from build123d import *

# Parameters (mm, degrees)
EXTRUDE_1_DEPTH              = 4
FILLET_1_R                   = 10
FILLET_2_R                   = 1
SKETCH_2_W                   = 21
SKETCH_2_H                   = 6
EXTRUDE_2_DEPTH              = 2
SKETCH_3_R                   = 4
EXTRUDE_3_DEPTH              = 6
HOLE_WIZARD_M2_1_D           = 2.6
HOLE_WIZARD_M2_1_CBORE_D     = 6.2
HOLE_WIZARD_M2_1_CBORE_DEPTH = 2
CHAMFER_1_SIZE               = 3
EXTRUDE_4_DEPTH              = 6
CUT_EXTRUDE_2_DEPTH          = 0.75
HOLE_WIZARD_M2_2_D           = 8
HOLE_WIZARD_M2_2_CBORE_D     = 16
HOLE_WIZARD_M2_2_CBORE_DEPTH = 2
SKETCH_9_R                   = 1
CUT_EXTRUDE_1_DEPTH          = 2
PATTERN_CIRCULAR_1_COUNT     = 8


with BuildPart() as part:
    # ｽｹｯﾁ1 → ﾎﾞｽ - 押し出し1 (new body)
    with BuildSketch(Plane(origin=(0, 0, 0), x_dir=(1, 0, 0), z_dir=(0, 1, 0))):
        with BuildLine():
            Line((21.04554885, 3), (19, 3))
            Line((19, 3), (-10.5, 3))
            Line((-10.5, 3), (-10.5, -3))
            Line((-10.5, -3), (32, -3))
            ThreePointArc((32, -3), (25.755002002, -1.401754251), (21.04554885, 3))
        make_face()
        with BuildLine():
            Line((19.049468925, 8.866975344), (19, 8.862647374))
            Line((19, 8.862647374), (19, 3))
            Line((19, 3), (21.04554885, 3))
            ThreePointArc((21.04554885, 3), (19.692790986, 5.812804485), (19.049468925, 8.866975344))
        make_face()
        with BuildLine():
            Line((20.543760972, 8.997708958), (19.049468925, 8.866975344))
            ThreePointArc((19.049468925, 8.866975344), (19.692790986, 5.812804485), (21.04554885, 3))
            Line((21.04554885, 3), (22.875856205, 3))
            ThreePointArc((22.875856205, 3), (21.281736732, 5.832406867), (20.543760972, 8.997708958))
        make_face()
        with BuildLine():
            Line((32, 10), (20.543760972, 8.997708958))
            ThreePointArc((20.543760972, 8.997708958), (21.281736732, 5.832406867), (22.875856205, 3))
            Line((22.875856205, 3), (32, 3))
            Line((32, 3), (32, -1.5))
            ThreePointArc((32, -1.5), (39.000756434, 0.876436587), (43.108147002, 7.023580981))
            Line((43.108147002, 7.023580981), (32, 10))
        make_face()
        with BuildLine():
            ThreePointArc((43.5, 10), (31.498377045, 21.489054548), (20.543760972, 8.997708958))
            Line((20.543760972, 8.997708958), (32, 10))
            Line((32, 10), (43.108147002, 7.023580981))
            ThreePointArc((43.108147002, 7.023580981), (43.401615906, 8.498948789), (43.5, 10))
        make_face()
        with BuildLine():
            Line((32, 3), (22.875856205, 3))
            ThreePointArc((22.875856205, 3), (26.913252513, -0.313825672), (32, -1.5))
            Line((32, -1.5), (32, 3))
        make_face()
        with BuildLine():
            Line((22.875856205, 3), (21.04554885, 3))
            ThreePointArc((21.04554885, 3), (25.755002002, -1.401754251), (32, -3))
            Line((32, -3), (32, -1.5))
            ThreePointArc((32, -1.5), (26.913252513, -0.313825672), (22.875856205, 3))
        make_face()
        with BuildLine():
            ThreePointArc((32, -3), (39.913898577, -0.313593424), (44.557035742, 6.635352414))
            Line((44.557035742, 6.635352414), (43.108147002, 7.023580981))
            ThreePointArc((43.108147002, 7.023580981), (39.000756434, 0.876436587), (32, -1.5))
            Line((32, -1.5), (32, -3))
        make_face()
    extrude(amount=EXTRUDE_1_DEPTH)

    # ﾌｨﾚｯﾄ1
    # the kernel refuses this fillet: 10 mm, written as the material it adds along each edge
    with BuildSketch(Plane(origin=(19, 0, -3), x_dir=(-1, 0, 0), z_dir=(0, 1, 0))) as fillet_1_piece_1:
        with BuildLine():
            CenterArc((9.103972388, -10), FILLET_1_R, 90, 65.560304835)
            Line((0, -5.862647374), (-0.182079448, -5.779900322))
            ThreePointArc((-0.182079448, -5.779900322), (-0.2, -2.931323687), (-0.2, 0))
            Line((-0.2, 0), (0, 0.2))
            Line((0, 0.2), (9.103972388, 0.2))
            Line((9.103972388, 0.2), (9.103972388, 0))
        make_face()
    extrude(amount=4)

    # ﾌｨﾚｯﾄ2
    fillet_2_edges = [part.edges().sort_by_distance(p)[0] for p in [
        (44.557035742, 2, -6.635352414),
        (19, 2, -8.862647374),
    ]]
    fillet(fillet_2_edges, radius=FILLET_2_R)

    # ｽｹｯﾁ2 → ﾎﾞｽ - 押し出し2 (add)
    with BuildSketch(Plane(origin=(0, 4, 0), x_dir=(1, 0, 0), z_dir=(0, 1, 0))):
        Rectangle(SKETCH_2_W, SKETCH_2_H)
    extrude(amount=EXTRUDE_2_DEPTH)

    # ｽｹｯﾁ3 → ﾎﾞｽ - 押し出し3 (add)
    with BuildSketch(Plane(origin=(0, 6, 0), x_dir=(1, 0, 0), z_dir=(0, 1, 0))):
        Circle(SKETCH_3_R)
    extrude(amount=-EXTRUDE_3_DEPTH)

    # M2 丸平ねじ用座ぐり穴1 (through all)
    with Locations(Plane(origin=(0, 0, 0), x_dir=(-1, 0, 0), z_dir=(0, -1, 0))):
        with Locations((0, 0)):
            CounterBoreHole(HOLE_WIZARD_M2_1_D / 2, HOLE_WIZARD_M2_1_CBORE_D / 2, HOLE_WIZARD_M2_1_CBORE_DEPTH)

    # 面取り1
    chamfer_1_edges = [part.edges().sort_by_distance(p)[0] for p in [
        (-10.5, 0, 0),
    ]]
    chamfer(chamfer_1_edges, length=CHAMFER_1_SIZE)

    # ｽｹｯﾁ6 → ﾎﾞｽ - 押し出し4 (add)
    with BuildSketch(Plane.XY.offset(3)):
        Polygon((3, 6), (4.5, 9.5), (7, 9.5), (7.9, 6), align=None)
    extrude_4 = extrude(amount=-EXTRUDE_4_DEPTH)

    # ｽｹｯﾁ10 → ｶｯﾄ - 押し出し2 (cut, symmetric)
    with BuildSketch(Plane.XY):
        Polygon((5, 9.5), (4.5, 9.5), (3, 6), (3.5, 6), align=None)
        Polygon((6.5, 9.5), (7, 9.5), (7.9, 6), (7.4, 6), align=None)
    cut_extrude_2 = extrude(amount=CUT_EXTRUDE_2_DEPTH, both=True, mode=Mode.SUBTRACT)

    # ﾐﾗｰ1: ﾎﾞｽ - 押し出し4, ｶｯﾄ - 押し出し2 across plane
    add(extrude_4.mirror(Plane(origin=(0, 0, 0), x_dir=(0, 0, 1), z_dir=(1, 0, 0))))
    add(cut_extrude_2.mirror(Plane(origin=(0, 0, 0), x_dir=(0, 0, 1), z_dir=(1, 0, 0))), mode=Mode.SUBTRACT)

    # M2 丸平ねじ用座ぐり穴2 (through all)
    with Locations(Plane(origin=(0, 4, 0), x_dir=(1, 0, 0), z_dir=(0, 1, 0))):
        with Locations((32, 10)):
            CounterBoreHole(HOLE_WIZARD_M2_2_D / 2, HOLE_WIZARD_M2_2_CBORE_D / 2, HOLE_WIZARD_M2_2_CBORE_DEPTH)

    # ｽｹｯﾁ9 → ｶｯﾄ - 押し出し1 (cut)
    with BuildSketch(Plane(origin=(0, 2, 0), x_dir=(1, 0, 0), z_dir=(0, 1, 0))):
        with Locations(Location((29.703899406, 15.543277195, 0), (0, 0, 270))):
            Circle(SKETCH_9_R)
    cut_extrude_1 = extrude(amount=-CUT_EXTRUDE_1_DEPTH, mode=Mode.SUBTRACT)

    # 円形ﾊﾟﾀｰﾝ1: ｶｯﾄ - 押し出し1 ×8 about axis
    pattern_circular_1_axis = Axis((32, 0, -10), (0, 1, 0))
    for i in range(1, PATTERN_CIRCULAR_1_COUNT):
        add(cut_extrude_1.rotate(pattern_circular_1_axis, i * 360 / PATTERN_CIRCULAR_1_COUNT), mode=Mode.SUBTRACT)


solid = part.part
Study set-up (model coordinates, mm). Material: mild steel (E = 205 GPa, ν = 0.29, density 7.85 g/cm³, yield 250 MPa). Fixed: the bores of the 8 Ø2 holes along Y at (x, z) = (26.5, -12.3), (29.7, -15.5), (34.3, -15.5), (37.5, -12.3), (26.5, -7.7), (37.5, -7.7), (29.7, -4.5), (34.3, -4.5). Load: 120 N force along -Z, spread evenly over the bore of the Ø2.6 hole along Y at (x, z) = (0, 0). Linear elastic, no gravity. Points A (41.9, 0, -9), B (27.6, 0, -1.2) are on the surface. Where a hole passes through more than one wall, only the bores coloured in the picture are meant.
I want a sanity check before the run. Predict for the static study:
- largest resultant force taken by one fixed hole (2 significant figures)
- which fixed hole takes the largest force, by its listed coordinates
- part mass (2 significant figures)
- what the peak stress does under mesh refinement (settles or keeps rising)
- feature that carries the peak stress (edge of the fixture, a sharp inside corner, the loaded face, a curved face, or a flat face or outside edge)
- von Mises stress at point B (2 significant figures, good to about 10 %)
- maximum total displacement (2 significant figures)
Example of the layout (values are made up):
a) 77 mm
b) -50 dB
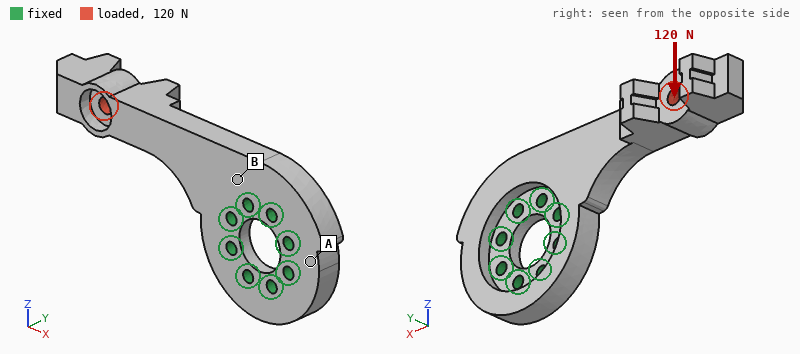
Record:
a) 170 N
b) (26.5, -12.3)
c) 20 g
d) keeps rising
e) a sharp inside corner
f) 20 MPa
g) 34 µm
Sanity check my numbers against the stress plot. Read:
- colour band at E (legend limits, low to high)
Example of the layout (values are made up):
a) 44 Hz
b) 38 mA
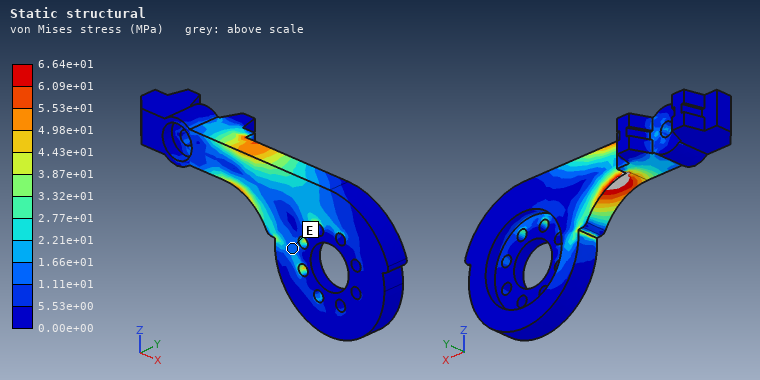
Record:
a) 1.11e+01 to 1.66e+01 MPa
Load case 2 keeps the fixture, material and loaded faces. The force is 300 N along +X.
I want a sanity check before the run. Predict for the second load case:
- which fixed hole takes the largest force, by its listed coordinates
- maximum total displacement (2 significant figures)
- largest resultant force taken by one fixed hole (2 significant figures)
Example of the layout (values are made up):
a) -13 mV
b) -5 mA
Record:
a) (29.7, -4.5)
b) 45 µm
c) 170 N
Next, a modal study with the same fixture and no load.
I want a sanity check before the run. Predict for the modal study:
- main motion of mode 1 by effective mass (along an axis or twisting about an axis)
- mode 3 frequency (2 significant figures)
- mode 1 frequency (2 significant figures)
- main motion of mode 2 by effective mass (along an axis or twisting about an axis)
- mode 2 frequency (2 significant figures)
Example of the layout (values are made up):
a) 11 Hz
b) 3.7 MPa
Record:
a) along Y
b) 10 kHz
c) 2000 Hz
d) along Z
e) 4600 Hz
